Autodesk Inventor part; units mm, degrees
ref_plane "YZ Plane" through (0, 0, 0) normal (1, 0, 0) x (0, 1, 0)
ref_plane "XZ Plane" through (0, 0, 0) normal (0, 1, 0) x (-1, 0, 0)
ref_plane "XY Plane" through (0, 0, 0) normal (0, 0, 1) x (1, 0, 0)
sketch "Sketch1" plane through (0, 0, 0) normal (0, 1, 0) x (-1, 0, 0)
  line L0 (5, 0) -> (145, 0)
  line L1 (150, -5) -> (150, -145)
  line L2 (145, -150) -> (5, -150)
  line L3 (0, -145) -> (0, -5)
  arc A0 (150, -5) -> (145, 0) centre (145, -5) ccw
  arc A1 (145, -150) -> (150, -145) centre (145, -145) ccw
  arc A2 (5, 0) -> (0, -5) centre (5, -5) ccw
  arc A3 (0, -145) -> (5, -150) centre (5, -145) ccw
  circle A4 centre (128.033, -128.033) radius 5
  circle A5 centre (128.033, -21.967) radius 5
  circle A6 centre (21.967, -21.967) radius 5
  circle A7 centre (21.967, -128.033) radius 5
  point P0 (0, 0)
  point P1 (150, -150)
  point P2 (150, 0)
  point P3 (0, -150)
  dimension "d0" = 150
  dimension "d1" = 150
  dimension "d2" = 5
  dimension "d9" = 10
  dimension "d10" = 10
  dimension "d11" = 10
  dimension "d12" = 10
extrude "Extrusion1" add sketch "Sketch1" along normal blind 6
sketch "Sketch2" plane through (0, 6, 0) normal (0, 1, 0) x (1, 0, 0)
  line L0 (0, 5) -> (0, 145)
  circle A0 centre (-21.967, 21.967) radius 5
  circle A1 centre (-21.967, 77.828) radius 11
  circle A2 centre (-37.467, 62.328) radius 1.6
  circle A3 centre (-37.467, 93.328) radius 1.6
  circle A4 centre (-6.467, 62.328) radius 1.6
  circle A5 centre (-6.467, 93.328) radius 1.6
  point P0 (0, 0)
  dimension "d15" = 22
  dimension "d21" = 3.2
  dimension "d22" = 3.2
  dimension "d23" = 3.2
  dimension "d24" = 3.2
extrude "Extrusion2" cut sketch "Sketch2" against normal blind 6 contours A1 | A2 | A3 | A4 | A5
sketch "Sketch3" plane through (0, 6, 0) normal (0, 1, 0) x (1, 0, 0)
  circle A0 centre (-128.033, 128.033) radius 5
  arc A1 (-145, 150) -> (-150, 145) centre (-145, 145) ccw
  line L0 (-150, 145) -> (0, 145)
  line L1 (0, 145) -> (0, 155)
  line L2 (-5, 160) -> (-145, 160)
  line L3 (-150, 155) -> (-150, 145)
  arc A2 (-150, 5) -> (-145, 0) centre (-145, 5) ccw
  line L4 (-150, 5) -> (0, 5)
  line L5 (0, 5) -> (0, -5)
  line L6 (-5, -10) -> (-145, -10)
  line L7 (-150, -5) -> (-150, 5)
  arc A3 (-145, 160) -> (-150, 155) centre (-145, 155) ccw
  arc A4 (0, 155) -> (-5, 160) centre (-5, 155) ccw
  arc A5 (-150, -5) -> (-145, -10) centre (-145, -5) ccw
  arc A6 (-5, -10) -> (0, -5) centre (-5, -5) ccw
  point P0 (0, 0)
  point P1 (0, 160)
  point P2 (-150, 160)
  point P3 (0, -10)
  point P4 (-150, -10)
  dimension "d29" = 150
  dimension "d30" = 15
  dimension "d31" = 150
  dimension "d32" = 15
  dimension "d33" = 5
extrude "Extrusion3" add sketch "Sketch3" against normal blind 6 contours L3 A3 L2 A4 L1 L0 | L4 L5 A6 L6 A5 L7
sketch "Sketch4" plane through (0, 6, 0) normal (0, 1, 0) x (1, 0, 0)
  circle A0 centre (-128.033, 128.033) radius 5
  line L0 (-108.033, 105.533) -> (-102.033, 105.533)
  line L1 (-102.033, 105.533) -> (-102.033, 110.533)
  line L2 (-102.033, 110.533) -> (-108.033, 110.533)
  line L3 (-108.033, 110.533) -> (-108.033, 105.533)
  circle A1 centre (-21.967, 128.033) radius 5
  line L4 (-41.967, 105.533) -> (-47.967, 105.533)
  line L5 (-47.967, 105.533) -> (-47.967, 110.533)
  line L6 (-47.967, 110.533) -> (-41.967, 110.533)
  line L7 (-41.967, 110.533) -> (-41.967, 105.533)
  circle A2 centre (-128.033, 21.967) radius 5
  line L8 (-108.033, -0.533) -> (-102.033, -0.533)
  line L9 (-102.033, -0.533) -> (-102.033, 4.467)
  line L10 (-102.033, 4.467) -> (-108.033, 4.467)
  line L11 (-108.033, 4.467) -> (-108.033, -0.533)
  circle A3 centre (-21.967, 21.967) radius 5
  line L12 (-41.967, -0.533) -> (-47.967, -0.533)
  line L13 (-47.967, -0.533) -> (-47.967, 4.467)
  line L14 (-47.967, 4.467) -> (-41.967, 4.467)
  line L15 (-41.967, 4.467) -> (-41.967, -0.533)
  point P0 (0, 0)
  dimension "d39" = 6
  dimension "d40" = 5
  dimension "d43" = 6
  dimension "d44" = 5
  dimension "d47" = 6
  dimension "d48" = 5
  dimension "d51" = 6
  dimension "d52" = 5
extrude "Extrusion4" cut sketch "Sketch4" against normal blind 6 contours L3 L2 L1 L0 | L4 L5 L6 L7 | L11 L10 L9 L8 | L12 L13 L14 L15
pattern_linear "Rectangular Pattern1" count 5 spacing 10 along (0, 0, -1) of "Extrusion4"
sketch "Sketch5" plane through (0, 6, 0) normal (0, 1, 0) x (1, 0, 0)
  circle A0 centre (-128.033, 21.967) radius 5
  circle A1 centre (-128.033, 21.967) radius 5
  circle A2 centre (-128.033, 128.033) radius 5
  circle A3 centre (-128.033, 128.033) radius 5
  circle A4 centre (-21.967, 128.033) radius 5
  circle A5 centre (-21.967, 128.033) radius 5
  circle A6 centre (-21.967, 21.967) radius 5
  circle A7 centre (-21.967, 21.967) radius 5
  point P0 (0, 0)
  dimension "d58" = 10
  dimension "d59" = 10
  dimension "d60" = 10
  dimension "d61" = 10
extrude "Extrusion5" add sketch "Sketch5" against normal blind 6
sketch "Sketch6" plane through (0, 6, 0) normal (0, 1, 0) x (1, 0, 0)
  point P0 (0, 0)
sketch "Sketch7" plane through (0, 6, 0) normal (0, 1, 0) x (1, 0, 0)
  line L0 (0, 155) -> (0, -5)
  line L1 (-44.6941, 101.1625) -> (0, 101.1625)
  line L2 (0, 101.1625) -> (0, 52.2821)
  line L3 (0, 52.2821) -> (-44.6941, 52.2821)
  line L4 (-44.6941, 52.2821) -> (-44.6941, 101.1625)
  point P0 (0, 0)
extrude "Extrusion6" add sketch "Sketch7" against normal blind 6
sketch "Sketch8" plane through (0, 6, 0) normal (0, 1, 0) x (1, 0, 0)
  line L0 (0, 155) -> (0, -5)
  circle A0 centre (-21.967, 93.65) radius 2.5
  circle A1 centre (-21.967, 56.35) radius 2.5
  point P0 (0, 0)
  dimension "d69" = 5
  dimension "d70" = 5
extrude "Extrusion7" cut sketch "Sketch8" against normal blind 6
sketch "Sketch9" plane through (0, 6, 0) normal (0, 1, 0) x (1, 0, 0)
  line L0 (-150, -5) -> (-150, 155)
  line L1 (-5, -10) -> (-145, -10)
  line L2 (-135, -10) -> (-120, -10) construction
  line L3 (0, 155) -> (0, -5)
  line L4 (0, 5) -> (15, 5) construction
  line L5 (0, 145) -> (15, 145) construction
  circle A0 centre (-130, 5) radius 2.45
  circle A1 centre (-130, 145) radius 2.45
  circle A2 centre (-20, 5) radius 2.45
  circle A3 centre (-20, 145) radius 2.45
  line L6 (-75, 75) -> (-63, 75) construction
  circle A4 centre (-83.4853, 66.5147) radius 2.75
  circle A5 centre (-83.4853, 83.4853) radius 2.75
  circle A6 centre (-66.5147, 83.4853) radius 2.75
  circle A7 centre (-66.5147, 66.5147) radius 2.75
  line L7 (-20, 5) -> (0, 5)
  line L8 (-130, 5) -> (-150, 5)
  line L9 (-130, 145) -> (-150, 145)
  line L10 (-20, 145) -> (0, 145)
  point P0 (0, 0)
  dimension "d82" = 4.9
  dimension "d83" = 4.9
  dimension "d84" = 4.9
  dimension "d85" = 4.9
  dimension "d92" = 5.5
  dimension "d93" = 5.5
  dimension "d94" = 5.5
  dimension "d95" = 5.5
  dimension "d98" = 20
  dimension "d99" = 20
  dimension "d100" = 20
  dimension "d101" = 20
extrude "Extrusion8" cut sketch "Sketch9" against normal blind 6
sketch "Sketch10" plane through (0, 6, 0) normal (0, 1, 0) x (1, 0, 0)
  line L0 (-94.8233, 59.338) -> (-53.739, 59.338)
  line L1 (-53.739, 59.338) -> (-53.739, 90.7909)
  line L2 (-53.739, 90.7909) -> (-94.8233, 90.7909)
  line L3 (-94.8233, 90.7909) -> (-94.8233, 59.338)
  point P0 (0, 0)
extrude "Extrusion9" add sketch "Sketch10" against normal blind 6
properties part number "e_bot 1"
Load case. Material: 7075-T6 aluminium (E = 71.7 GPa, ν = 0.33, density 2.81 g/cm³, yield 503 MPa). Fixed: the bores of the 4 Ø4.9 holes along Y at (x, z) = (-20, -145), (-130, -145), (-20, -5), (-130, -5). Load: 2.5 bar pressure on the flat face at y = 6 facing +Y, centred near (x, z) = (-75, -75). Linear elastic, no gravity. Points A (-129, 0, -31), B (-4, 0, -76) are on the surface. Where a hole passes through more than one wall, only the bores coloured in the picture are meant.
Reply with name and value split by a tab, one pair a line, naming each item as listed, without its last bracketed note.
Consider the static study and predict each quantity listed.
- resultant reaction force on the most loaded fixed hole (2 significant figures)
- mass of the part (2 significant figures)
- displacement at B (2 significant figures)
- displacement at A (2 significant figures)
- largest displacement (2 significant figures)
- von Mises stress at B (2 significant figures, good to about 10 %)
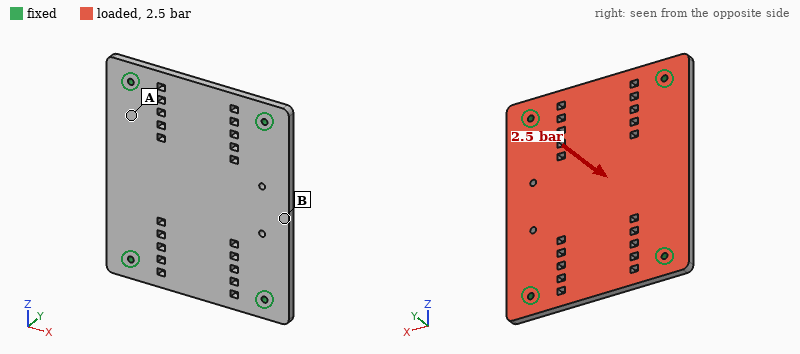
resultant reaction force on the most loaded fixed hole	1.6 kN
mass of the part	420 g
displacement at B	0.27 mm
displacement at A	0.13 mm
largest displacement	0.37 mm
von Mises stress at B	45 MPa
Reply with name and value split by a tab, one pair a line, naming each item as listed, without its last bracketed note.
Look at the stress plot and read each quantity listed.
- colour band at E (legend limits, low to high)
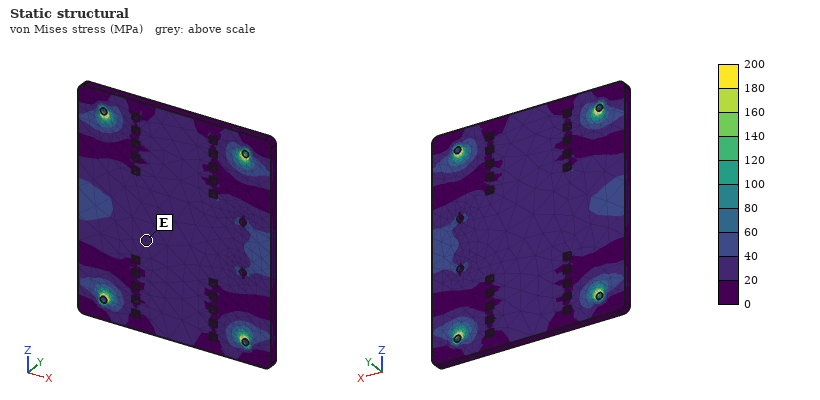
colour band at E	20 to 40 MPa
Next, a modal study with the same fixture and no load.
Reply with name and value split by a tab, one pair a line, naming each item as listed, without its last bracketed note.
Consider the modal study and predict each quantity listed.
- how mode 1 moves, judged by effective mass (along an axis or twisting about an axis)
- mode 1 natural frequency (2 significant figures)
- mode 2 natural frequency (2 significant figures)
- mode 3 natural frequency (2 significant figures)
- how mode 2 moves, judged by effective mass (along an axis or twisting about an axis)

how mode 1 moves, judged by effective mass	along Y
mode 1 natural frequency	1200 Hz
mode 2 natural frequency	1700 Hz
mode 3 natural frequency	2200 Hz
how mode 2 moves, judged by effective mass	twisting about Z
